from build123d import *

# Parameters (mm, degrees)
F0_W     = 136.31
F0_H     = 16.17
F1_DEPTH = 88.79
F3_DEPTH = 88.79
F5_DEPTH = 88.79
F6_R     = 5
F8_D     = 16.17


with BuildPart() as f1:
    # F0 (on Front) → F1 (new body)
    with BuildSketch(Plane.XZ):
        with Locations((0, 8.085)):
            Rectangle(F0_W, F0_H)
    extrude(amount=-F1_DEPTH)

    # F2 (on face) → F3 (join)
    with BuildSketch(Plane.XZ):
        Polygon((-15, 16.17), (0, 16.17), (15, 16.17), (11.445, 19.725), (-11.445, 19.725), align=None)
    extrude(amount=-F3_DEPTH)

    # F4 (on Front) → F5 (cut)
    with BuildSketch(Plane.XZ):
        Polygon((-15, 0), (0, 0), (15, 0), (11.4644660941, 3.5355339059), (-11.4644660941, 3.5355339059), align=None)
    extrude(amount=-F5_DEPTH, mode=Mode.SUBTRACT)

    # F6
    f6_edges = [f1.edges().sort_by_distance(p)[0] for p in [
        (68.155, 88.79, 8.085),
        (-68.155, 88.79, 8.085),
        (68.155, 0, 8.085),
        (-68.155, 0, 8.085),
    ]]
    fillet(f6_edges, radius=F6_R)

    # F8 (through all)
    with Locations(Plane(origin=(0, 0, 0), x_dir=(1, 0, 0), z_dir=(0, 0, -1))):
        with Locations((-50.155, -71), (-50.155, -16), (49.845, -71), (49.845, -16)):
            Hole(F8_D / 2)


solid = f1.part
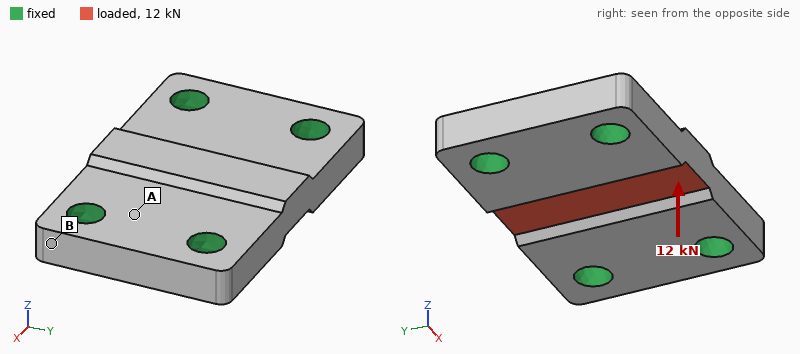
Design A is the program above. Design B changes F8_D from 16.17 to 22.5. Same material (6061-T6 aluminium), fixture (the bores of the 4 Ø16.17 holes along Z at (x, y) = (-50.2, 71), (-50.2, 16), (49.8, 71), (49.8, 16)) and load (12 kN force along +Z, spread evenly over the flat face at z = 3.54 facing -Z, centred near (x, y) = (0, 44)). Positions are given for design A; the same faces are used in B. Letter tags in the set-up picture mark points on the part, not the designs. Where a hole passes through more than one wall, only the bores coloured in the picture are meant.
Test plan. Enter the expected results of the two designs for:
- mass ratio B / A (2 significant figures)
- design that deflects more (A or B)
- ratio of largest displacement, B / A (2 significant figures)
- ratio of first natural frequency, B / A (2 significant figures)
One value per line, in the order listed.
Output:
0.93
A
0.79
1.2
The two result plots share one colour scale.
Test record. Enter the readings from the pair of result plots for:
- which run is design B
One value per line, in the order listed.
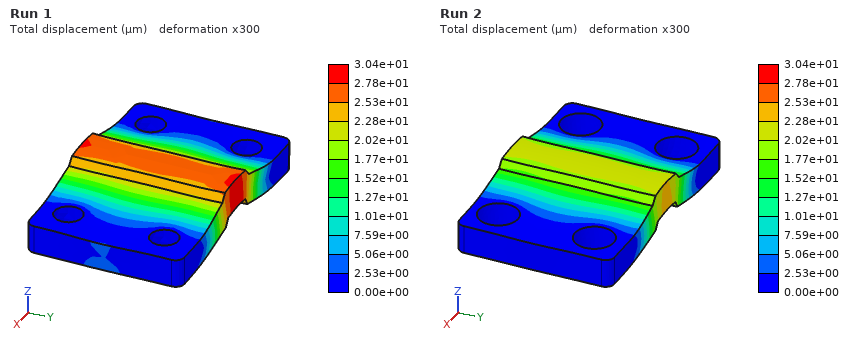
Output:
Run 2
